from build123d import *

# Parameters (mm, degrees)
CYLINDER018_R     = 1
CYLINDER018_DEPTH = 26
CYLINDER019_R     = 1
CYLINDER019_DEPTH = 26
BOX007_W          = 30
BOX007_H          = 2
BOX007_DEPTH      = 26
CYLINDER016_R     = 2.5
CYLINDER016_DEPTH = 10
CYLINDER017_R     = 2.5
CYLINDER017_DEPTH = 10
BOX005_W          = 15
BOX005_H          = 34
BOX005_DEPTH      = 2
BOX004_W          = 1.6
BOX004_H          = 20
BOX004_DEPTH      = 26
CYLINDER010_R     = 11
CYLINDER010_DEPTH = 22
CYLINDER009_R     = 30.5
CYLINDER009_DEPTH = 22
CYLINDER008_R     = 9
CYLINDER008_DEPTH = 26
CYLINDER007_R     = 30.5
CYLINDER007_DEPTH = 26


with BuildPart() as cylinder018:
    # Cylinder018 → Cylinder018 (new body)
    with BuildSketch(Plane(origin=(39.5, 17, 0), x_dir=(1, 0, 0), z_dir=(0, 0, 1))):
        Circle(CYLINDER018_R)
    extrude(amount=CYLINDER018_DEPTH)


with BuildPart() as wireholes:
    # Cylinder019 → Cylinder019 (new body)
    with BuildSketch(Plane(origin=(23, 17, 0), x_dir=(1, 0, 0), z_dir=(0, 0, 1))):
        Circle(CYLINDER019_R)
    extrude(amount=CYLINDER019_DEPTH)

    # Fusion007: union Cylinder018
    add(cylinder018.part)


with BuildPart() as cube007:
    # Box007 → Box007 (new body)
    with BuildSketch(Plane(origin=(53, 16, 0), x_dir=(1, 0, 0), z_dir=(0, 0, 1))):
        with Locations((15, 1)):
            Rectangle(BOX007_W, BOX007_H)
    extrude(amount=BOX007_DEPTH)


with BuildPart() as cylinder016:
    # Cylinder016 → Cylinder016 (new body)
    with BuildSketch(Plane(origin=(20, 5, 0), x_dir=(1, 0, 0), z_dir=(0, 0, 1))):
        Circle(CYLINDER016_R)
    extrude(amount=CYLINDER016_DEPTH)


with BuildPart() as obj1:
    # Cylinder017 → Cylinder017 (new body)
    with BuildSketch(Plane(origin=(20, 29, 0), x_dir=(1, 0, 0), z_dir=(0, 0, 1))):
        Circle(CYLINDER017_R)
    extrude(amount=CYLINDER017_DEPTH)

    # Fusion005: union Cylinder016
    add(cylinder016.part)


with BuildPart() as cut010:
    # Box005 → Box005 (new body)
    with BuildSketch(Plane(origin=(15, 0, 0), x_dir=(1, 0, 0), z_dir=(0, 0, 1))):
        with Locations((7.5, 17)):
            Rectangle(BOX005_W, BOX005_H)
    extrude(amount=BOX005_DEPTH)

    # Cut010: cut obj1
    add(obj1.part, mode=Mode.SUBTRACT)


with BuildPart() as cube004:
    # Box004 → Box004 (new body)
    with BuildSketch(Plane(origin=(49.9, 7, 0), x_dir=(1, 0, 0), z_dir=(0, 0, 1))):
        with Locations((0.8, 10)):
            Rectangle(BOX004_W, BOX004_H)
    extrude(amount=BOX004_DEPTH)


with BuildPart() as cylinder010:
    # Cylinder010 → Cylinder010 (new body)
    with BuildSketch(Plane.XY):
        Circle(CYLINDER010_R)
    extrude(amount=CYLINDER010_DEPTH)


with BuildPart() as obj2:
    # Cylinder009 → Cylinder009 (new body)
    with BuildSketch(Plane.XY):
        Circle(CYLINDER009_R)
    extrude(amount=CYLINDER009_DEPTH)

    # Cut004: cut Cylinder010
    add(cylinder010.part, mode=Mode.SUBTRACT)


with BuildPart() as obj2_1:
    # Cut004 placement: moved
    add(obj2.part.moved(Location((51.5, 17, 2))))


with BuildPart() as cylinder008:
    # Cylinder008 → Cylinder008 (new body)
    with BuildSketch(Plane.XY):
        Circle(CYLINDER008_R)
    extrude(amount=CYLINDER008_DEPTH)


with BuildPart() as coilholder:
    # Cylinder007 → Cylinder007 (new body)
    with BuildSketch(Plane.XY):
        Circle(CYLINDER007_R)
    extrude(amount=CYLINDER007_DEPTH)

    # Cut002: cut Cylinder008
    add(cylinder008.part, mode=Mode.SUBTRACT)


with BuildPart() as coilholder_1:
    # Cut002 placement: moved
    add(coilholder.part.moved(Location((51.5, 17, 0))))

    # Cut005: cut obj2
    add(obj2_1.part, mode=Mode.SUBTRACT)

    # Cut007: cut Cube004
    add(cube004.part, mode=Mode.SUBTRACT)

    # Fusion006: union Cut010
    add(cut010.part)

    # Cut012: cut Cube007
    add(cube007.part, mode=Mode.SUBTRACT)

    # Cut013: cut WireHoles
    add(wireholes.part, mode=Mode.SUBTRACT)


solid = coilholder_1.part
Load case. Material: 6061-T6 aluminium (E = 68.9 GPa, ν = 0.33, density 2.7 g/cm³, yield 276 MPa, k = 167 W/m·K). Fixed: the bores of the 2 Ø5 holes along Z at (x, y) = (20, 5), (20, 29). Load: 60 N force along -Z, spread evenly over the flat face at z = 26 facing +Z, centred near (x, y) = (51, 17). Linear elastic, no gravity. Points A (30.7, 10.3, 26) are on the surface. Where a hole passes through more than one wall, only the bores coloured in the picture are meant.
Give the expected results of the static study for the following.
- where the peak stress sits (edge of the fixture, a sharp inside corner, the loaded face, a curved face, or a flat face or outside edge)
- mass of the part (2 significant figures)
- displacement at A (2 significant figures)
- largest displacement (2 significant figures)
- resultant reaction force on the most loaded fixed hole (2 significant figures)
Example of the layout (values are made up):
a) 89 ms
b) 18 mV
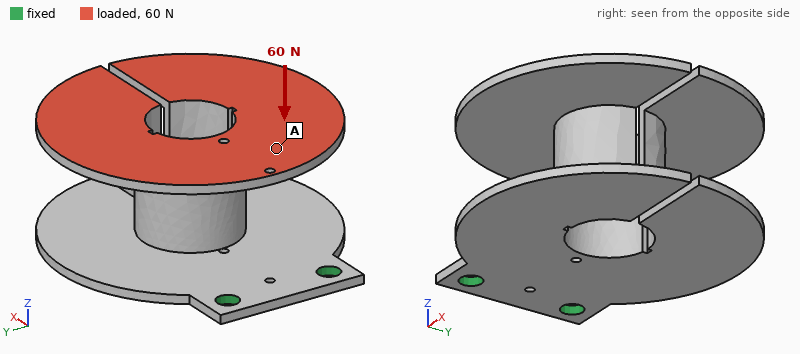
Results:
a) a flat face or outside edge
b) 36 g
c) 0.34 mm
d) 0.82 mm
e) 30 N
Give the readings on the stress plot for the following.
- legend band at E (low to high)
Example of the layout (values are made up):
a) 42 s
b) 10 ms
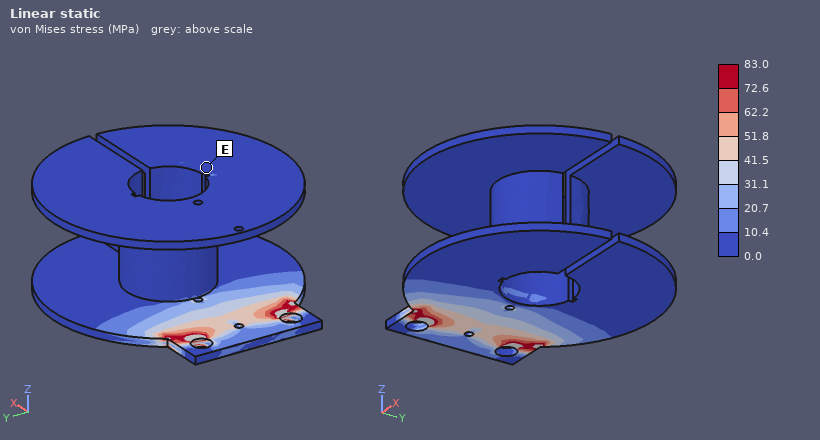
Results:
a) 0.0 to 10.4 MPa
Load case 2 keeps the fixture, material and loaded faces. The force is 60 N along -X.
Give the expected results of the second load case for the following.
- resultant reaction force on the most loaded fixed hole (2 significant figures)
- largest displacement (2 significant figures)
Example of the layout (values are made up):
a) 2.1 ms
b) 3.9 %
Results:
a) 30 N
b) 1.0 mm
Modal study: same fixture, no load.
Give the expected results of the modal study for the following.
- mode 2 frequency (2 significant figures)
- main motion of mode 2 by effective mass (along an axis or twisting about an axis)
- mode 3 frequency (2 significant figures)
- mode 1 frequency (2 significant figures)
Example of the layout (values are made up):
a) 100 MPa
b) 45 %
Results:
a) 610 Hz
b) along Y
c) 780 Hz
d) 260 Hz
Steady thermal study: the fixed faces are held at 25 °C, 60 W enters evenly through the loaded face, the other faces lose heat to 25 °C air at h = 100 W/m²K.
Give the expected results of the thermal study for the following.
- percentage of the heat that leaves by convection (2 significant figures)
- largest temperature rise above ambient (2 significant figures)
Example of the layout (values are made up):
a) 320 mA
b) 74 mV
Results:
a) 79 %
b) 76 K
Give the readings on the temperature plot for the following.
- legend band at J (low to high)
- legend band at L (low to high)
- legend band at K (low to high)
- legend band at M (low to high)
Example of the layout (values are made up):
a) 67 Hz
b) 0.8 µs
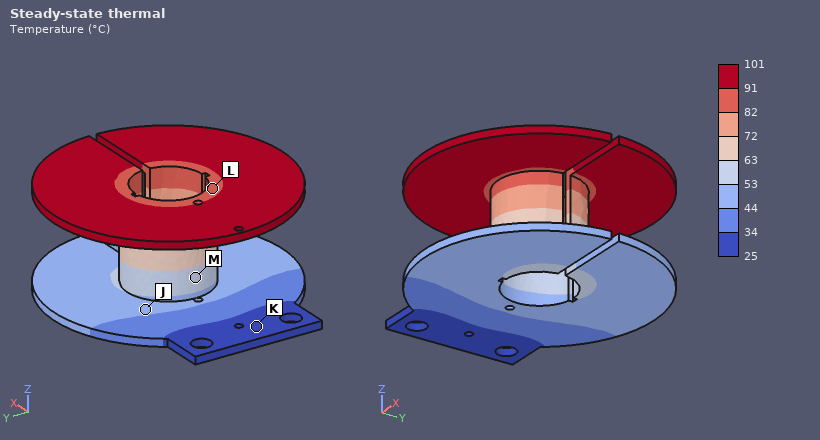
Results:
a) 44 to 53 °C
b) 82 to 91 °C
c) 25 to 34 °C
d) 53 to 63 °C
